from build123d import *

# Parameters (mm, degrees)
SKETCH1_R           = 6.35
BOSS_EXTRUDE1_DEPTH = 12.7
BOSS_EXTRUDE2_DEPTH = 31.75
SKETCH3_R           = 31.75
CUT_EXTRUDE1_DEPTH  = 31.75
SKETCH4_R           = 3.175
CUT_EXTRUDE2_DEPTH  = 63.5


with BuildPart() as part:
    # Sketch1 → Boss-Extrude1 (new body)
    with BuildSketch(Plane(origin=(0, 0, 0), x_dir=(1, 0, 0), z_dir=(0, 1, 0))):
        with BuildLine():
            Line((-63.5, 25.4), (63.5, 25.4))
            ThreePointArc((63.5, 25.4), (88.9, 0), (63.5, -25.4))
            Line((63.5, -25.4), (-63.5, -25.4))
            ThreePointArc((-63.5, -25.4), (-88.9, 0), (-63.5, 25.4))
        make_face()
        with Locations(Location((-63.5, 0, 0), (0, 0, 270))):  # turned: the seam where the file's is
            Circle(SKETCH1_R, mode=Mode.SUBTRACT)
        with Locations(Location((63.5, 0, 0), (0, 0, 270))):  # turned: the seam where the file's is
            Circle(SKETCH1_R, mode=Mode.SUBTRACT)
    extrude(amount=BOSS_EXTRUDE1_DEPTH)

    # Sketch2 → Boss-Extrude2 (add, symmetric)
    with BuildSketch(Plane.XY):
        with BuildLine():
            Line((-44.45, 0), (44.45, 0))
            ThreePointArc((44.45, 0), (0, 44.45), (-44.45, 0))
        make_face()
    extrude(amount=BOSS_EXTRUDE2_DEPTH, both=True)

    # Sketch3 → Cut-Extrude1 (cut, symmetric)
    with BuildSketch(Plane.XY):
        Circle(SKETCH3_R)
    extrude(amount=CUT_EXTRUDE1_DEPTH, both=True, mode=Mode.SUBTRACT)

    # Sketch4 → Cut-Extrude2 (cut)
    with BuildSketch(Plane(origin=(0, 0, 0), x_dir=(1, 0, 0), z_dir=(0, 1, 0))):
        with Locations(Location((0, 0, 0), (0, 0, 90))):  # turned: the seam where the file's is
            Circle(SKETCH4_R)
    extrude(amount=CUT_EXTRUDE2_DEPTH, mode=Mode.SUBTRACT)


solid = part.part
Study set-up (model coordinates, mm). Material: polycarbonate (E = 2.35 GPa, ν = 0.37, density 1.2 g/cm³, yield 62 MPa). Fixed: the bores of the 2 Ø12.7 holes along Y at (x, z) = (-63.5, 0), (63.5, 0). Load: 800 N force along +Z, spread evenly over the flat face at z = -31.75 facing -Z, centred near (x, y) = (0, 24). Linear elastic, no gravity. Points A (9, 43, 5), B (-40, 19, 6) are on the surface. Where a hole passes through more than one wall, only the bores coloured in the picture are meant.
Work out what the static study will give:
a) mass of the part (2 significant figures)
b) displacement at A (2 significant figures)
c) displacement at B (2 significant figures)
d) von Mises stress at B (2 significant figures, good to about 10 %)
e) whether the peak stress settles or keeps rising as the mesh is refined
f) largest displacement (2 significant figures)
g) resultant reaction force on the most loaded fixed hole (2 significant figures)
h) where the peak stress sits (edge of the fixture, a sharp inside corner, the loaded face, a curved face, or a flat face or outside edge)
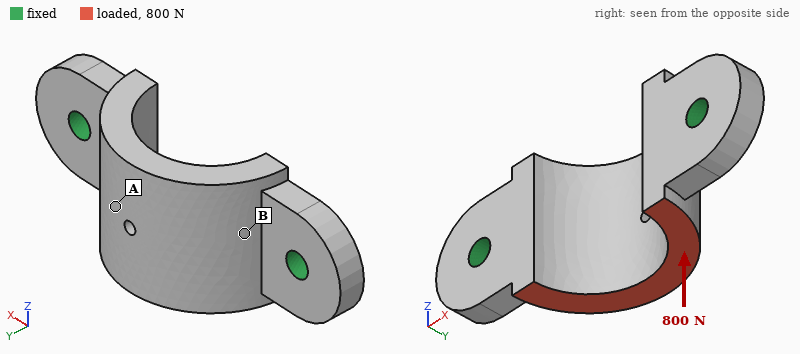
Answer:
170 g
0.32 mm
0.14 mm
2.6 MPa
keeps rising
0.40 mm
400 N
edge of the fixture
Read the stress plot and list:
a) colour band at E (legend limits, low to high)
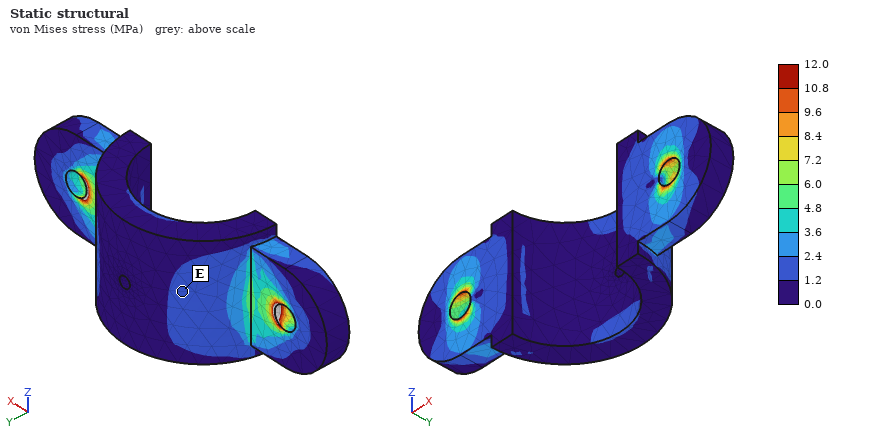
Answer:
1.2 to 2.4 MPa
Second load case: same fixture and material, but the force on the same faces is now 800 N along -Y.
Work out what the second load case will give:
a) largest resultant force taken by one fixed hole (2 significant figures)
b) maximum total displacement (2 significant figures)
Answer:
510 N
0.57 mm
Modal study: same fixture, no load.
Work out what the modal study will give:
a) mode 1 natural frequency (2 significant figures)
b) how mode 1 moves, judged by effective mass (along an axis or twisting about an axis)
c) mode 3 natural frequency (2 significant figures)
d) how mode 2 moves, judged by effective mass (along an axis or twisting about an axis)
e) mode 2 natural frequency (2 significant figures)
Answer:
750 Hz
along Z
1900 Hz
along Y
1600 Hz
